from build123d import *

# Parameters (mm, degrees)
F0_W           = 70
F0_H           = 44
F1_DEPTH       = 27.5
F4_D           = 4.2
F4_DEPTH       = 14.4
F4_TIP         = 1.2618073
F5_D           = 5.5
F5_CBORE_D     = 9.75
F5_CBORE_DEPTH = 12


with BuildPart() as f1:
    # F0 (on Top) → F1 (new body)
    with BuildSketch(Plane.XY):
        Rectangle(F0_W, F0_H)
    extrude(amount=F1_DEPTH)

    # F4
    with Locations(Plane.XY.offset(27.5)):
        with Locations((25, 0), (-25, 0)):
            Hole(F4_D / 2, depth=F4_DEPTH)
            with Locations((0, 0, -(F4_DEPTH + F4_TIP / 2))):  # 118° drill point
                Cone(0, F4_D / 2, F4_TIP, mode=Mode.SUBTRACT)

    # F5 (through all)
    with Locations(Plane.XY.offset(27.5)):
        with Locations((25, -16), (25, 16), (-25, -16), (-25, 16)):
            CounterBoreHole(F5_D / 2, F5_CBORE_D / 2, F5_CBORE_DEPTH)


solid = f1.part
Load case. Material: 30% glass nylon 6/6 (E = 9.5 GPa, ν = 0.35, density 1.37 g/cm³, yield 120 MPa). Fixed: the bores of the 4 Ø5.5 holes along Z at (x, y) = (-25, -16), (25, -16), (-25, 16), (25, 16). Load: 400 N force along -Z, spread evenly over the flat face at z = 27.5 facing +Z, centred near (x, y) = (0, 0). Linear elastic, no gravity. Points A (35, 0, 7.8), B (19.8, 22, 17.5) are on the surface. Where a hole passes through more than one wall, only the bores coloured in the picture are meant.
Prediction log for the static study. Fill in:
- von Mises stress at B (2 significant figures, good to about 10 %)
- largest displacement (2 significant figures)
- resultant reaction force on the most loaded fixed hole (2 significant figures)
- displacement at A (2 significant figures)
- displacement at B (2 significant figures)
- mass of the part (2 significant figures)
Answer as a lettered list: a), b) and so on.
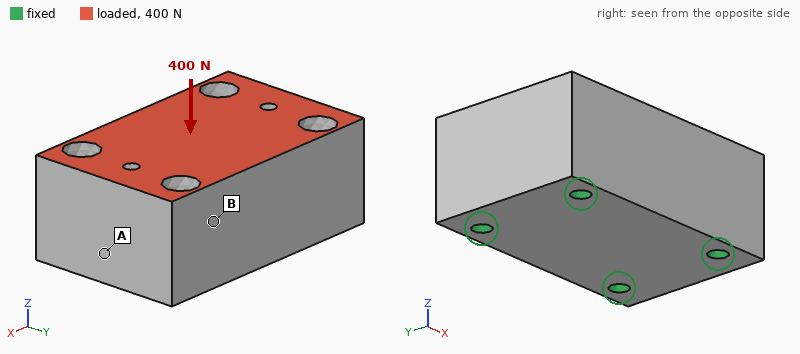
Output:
a) 0.34 MPa
b) 1.2 µm
c) 100 N
d) 0.46 µm
e) 0.56 µm
f) 110 g
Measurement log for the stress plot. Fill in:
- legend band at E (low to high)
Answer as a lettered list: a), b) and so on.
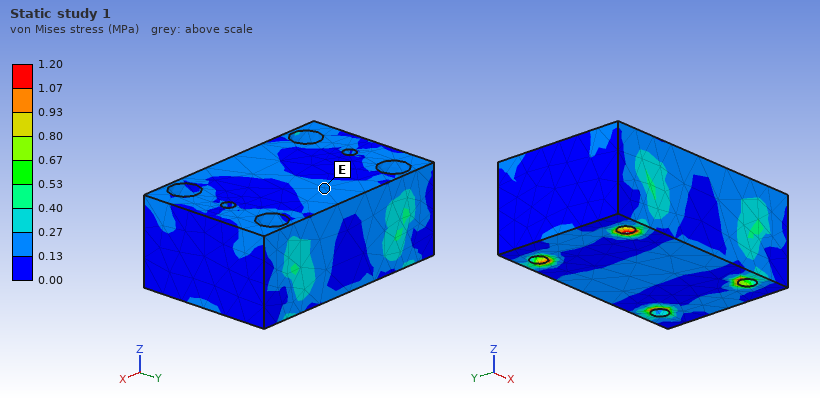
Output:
a) 0.13 to 0.27 MPa
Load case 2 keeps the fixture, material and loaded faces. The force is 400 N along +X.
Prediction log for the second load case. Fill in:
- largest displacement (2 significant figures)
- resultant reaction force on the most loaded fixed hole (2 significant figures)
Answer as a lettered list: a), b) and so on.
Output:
a) 2.3 µm
b) 120 N
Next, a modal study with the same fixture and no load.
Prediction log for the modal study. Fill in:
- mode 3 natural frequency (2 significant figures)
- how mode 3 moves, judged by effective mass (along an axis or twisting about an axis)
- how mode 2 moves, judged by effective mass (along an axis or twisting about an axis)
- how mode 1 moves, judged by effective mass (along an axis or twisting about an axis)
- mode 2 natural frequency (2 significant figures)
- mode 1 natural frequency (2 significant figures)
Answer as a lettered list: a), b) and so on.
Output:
a) 13 kHz
b) along X
c) along Y
d) along Z
e) 11 kHz
f) 10 kHz
